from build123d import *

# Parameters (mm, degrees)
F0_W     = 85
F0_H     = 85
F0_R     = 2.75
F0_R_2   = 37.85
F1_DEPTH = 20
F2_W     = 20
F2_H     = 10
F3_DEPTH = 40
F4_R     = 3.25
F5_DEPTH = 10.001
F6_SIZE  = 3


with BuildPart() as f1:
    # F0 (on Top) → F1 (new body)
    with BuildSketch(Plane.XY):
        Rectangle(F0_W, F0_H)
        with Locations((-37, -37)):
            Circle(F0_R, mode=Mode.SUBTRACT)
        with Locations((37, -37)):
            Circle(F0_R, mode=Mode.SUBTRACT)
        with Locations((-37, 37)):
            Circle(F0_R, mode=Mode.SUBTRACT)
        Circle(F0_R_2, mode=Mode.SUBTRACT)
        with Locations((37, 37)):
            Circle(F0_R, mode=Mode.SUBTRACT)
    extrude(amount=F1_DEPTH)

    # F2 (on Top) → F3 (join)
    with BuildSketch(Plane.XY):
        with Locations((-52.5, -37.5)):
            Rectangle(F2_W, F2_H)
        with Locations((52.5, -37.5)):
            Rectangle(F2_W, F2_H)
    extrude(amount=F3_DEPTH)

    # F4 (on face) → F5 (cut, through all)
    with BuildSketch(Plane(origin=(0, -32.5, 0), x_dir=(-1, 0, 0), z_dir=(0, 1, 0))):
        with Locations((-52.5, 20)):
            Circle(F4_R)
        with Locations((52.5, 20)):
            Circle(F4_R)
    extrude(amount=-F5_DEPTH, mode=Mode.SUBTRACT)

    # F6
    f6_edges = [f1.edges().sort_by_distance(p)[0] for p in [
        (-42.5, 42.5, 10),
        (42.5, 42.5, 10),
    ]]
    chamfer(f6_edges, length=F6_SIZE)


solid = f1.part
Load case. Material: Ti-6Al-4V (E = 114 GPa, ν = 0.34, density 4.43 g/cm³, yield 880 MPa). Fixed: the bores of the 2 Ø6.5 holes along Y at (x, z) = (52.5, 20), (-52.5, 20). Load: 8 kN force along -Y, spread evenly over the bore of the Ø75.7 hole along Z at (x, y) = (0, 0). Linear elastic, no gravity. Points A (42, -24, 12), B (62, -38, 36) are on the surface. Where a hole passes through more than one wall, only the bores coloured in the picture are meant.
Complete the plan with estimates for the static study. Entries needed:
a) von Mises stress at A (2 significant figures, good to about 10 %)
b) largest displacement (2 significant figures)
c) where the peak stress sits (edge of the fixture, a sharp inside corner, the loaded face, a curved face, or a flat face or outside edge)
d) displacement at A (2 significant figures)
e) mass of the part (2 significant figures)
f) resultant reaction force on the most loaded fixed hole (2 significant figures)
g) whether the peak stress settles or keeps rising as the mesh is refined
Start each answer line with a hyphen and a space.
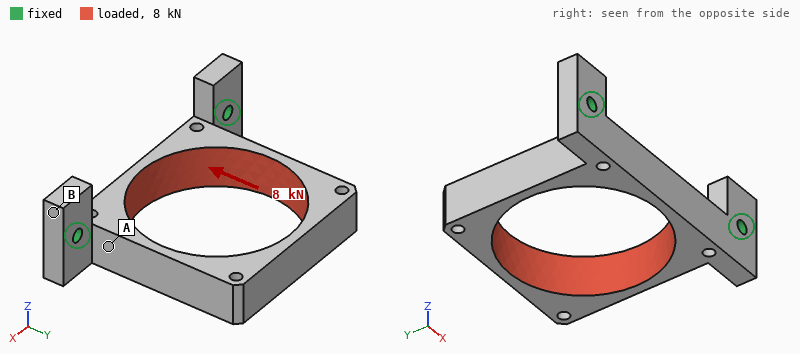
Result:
- 67 MPa
- 0.14 mm
- edge of the fixture
- 0.041 mm
- 300 g
- 4.0 kN
- keeps rising
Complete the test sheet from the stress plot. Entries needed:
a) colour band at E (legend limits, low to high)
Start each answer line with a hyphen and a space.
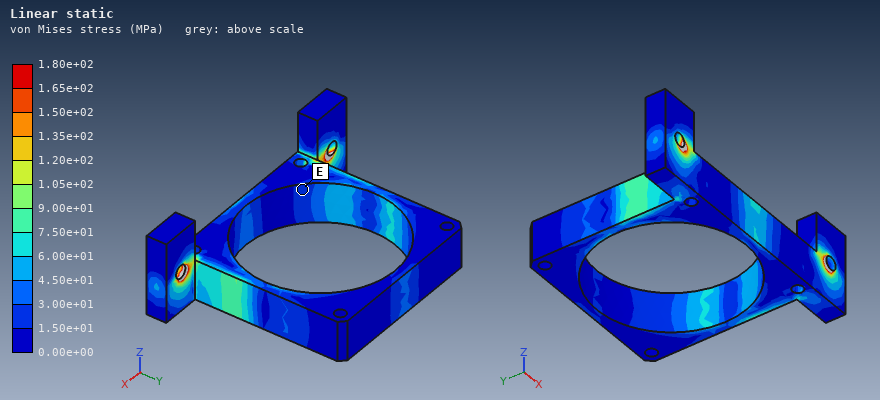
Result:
- 1.50e+01 to 3.00e+01 MPa
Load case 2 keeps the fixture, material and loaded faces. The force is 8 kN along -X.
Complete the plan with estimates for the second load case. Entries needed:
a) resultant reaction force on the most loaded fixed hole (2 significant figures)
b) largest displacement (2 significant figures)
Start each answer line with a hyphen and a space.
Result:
- 4.9 kN
- 0.45 mm
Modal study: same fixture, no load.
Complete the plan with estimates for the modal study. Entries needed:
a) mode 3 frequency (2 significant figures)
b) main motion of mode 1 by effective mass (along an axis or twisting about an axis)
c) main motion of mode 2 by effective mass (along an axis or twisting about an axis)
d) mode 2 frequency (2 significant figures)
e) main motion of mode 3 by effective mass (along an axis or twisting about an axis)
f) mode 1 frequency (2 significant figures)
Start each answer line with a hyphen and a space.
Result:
- 1800 Hz
- along Z
- along X
- 1500 Hz
- twisting about Y
- 930 Hz
